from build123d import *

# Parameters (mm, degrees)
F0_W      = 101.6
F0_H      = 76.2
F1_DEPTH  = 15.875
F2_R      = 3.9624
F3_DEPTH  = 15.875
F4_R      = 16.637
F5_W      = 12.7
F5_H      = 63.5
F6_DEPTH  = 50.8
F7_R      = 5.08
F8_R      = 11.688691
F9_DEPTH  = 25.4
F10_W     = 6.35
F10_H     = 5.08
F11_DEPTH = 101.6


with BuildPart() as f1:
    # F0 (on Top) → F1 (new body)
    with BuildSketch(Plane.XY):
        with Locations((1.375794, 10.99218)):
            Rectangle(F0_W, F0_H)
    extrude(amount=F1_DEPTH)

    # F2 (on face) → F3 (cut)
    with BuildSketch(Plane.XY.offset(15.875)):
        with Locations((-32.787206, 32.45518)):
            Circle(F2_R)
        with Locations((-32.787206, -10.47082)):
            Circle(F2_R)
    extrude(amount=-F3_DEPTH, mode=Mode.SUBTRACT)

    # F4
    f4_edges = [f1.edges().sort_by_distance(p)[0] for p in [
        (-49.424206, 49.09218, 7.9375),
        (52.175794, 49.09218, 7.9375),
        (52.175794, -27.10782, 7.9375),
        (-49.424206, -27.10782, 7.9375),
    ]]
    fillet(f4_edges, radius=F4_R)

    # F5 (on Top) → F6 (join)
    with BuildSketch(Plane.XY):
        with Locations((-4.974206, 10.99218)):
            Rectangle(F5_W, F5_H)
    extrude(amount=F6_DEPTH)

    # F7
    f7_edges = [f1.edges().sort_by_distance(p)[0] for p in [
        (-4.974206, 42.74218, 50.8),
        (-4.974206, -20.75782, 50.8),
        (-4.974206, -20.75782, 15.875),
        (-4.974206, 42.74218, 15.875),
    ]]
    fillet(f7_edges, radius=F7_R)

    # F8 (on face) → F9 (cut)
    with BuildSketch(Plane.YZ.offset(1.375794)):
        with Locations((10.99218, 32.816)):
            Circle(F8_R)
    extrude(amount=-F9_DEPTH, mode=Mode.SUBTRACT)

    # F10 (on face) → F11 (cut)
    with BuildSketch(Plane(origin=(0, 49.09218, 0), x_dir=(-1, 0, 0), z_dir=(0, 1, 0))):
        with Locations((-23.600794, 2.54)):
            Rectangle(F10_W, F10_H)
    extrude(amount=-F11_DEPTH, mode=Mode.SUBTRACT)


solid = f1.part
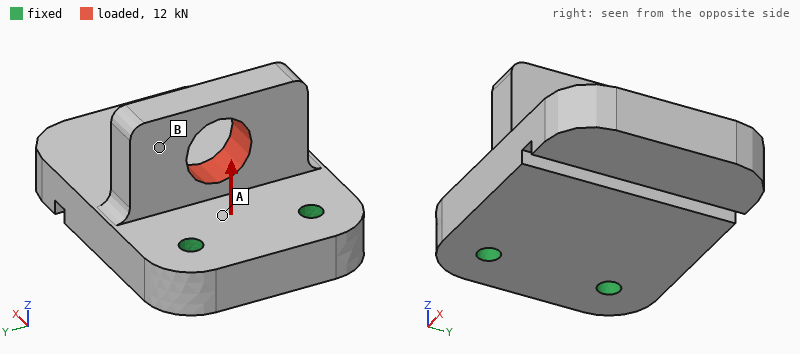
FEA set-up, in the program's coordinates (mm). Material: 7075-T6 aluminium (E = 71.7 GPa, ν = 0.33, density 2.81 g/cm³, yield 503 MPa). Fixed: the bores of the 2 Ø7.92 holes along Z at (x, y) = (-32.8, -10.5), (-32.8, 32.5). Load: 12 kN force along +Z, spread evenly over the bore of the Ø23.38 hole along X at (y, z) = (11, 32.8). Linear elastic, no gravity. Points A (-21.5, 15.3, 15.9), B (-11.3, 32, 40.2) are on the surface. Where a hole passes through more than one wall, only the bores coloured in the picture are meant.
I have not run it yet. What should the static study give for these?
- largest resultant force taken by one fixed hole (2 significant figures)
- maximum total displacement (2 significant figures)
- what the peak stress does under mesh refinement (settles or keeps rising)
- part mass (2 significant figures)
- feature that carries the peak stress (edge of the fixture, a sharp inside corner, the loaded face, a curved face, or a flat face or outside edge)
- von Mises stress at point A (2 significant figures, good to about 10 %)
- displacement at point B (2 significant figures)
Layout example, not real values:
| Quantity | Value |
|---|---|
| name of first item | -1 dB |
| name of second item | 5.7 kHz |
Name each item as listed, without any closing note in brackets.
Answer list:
| Quantity | Value |
|---|---|
| largest resultant force taken by one fixed hole | 6.0 kN |
| maximum total displacement | 0.24 mm |
| what the peak stress does under mesh refinement | keeps rising |
| part mass | 390 g |
| feature that carries the peak stress | edge of the fixture |
| von Mises stress at point A | 40 MPa |
| displacement at point B | 0.11 mm |
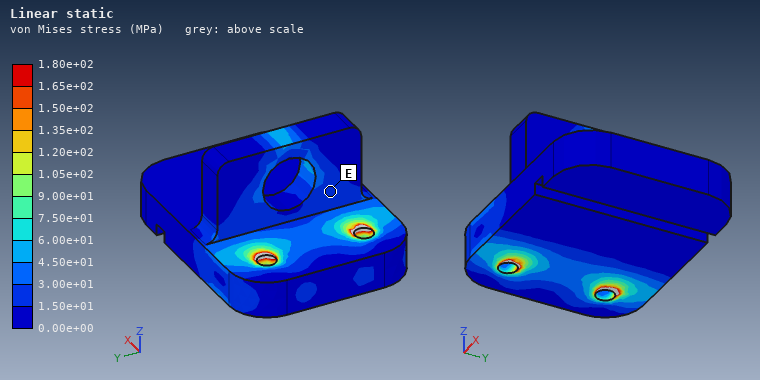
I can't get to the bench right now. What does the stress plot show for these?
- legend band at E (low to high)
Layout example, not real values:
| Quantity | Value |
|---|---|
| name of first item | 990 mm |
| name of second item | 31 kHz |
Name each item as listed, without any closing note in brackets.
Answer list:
| Quantity | Value |
|---|---|
| legend band at E | 1.50e+01 to 3.00e+01 MPa |
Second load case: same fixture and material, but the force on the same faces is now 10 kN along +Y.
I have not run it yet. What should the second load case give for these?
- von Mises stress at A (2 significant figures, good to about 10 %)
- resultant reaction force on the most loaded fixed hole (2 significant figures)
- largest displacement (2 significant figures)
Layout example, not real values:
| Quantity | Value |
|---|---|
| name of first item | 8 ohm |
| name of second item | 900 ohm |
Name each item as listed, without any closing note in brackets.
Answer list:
| Quantity | Value |
|---|---|
| von Mises stress at A | 44 MPa |
| resultant reaction force on the most loaded fixed hole | 8.8 kN |
| largest displacement | 95 µm |
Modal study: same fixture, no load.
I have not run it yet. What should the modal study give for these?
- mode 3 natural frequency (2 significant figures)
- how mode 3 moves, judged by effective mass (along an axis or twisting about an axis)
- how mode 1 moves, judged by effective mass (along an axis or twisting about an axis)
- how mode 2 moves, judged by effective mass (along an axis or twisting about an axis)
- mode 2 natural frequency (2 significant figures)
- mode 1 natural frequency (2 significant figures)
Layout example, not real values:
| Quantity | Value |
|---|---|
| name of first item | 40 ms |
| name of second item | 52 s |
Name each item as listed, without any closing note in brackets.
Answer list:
| Quantity | Value |
|---|---|
| mode 3 natural frequency | 5200 Hz |
| how mode 3 moves, judged by effective mass | along Y |
| how mode 1 moves, judged by effective mass | along Z |
| how mode 2 moves, judged by effective mass | twisting about X |
| mode 2 natural frequency | 4200 Hz |
| mode 1 natural frequency | 1700 Hz |
